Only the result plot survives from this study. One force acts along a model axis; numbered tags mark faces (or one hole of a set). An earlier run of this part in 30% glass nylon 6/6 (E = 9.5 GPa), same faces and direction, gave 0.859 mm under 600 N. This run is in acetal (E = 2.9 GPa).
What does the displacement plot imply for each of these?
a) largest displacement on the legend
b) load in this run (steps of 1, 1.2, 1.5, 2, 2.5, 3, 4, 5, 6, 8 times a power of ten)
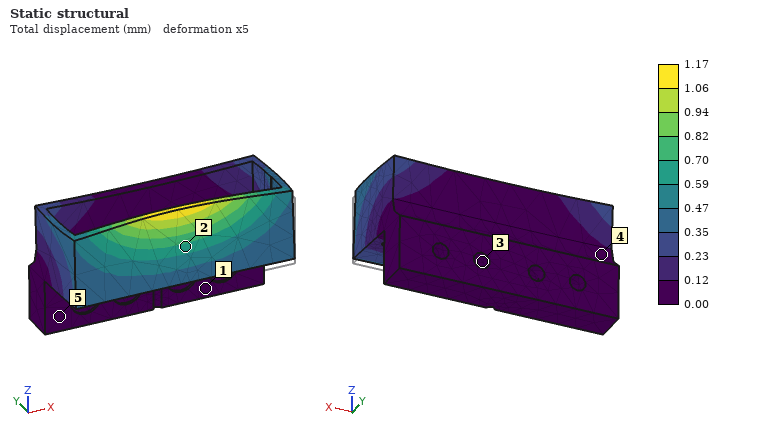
1.17 mm
250 N
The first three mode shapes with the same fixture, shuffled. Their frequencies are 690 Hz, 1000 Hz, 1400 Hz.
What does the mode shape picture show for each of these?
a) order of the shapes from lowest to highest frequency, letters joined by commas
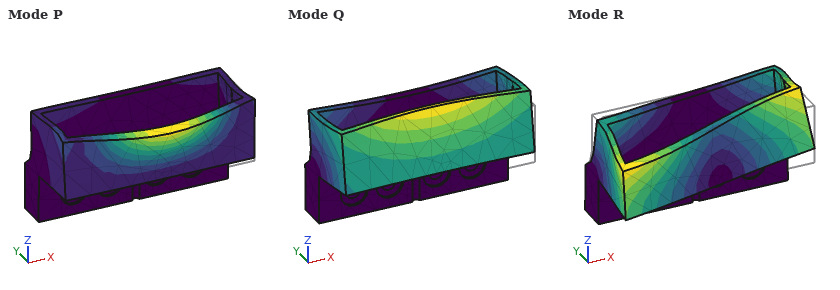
Q, R, P
